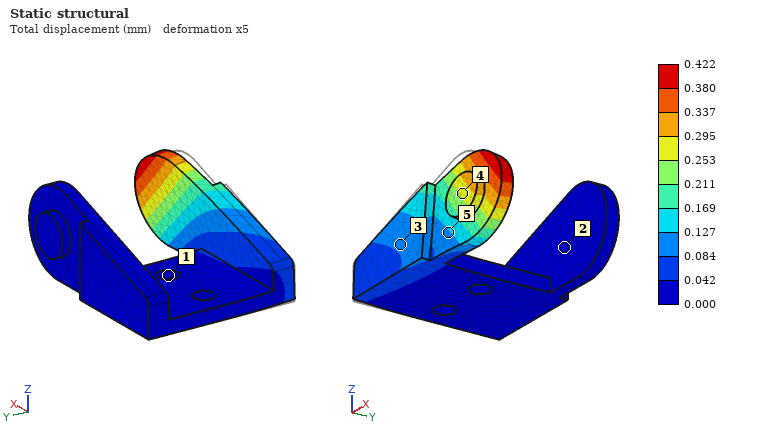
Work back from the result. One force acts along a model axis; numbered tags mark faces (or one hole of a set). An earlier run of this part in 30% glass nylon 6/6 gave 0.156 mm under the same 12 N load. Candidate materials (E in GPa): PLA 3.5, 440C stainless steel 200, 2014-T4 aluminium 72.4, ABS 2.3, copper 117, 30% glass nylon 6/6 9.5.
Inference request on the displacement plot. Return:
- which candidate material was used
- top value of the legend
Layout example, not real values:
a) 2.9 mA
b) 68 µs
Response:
a) PLA
b) 0.422 mm
